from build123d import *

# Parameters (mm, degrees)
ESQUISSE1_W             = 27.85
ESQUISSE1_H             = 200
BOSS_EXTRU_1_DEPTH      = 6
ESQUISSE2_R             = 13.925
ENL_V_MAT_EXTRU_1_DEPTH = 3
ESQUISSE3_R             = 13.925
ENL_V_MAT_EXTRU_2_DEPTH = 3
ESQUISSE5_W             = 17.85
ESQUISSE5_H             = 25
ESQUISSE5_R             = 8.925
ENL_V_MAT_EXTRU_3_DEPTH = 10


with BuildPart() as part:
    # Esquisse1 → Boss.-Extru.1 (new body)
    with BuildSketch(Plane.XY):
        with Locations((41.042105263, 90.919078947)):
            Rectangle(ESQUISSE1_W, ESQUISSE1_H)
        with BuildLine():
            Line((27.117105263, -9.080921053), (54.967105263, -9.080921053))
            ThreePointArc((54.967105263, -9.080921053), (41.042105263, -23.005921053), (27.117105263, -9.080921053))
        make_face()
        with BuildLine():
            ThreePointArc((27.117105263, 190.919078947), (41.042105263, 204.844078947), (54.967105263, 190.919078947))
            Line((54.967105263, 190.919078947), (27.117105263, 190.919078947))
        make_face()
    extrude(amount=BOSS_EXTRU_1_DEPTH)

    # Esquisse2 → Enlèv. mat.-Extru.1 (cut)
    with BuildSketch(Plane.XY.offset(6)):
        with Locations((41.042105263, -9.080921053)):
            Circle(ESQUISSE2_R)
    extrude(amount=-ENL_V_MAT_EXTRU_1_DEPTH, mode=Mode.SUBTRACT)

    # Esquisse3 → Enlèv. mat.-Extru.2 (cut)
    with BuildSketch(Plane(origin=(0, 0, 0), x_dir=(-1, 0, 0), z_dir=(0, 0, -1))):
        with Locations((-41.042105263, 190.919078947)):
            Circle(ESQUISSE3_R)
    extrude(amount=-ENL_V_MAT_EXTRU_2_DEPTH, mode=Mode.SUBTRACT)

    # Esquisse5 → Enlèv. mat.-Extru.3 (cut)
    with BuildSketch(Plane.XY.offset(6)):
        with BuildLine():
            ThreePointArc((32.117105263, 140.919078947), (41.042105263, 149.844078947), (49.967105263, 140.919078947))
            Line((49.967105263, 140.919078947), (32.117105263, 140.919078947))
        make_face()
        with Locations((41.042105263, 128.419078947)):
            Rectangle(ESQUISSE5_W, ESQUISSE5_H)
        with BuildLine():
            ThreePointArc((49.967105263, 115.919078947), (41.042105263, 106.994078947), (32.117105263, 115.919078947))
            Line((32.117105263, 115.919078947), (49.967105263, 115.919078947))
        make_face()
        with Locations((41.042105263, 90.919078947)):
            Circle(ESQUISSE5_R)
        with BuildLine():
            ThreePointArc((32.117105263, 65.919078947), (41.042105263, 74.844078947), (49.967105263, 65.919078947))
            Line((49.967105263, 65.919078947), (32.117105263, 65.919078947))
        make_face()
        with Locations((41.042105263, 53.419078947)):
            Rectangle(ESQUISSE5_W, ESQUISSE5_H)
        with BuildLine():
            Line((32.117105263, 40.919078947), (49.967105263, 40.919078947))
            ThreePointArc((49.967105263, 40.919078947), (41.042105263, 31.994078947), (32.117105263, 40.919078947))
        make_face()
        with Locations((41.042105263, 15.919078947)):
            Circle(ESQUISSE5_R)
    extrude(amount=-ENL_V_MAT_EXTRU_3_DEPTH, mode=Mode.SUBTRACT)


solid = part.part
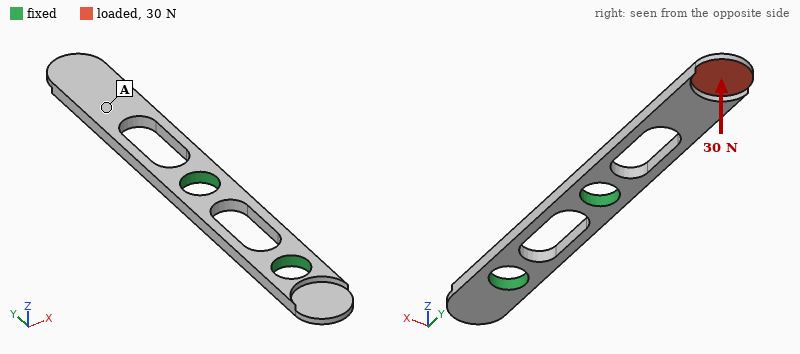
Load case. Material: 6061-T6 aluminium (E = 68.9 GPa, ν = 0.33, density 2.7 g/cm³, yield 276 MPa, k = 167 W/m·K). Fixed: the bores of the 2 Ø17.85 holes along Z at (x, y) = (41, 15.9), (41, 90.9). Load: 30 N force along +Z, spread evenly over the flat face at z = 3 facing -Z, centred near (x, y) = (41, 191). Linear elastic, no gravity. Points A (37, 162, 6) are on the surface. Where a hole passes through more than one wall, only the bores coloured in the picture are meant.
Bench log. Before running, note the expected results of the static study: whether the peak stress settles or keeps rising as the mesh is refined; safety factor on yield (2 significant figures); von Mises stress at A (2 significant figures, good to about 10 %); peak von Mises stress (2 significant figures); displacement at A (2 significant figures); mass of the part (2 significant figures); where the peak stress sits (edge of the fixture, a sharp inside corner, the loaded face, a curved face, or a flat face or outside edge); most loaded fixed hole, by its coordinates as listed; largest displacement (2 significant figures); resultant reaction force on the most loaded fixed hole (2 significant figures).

settles
6.3
5.3 MPa
44 MPa
0.27 mm
60 g
a curved face
(41, 90.9)
0.61 mm
30 N
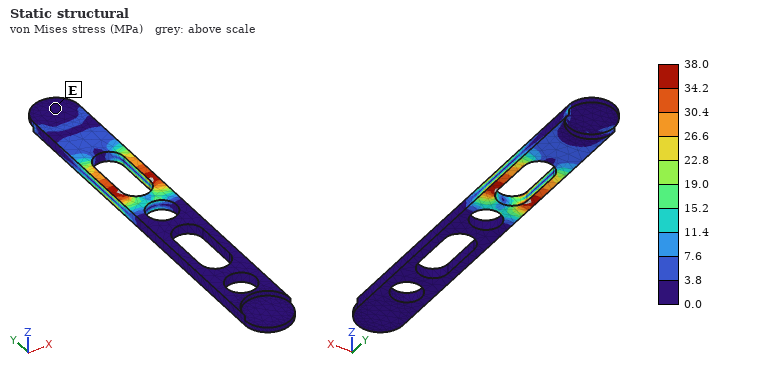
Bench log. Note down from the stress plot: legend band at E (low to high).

0.0 to 3.8 MPa
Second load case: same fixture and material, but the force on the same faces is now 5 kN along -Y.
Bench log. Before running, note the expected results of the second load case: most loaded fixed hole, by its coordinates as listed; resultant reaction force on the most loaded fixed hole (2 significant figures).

(41, 90.9)
5.0 kN
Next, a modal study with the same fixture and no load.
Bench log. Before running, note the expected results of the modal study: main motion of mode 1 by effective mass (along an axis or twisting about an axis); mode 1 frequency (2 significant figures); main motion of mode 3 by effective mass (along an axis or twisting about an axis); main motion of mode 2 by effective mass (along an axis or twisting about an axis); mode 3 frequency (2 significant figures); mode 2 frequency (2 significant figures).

along Z
380 Hz
twisting about Y
along X
2100 Hz
1200 Hz
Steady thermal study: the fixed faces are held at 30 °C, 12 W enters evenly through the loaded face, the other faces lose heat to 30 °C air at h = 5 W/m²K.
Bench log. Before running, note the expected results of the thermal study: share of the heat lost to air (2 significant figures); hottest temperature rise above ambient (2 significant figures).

9.8 %
71 K
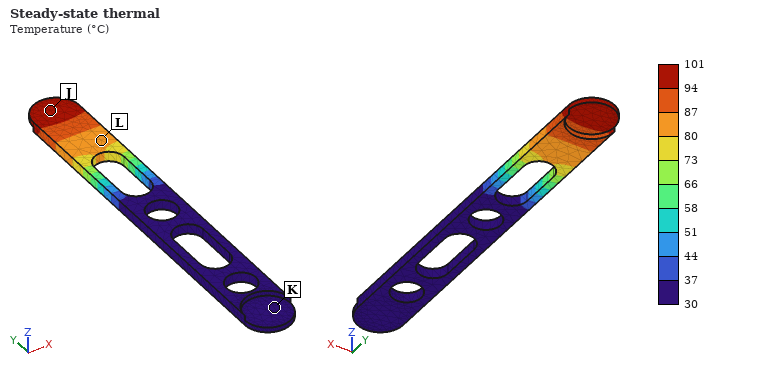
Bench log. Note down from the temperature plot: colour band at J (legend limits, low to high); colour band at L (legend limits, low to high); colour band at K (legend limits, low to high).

94 to 101 °C
80 to 87 °C
30 to 37 °C
